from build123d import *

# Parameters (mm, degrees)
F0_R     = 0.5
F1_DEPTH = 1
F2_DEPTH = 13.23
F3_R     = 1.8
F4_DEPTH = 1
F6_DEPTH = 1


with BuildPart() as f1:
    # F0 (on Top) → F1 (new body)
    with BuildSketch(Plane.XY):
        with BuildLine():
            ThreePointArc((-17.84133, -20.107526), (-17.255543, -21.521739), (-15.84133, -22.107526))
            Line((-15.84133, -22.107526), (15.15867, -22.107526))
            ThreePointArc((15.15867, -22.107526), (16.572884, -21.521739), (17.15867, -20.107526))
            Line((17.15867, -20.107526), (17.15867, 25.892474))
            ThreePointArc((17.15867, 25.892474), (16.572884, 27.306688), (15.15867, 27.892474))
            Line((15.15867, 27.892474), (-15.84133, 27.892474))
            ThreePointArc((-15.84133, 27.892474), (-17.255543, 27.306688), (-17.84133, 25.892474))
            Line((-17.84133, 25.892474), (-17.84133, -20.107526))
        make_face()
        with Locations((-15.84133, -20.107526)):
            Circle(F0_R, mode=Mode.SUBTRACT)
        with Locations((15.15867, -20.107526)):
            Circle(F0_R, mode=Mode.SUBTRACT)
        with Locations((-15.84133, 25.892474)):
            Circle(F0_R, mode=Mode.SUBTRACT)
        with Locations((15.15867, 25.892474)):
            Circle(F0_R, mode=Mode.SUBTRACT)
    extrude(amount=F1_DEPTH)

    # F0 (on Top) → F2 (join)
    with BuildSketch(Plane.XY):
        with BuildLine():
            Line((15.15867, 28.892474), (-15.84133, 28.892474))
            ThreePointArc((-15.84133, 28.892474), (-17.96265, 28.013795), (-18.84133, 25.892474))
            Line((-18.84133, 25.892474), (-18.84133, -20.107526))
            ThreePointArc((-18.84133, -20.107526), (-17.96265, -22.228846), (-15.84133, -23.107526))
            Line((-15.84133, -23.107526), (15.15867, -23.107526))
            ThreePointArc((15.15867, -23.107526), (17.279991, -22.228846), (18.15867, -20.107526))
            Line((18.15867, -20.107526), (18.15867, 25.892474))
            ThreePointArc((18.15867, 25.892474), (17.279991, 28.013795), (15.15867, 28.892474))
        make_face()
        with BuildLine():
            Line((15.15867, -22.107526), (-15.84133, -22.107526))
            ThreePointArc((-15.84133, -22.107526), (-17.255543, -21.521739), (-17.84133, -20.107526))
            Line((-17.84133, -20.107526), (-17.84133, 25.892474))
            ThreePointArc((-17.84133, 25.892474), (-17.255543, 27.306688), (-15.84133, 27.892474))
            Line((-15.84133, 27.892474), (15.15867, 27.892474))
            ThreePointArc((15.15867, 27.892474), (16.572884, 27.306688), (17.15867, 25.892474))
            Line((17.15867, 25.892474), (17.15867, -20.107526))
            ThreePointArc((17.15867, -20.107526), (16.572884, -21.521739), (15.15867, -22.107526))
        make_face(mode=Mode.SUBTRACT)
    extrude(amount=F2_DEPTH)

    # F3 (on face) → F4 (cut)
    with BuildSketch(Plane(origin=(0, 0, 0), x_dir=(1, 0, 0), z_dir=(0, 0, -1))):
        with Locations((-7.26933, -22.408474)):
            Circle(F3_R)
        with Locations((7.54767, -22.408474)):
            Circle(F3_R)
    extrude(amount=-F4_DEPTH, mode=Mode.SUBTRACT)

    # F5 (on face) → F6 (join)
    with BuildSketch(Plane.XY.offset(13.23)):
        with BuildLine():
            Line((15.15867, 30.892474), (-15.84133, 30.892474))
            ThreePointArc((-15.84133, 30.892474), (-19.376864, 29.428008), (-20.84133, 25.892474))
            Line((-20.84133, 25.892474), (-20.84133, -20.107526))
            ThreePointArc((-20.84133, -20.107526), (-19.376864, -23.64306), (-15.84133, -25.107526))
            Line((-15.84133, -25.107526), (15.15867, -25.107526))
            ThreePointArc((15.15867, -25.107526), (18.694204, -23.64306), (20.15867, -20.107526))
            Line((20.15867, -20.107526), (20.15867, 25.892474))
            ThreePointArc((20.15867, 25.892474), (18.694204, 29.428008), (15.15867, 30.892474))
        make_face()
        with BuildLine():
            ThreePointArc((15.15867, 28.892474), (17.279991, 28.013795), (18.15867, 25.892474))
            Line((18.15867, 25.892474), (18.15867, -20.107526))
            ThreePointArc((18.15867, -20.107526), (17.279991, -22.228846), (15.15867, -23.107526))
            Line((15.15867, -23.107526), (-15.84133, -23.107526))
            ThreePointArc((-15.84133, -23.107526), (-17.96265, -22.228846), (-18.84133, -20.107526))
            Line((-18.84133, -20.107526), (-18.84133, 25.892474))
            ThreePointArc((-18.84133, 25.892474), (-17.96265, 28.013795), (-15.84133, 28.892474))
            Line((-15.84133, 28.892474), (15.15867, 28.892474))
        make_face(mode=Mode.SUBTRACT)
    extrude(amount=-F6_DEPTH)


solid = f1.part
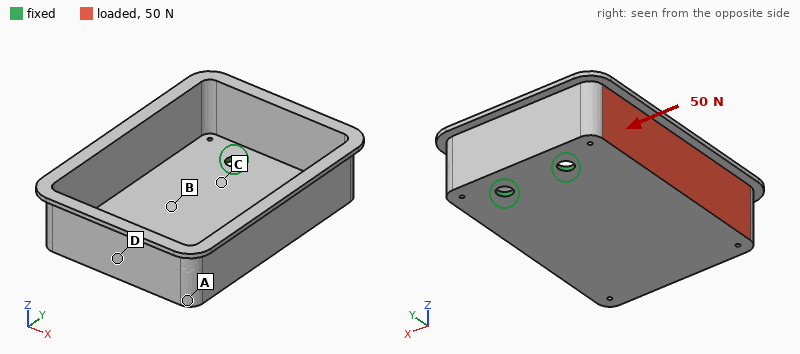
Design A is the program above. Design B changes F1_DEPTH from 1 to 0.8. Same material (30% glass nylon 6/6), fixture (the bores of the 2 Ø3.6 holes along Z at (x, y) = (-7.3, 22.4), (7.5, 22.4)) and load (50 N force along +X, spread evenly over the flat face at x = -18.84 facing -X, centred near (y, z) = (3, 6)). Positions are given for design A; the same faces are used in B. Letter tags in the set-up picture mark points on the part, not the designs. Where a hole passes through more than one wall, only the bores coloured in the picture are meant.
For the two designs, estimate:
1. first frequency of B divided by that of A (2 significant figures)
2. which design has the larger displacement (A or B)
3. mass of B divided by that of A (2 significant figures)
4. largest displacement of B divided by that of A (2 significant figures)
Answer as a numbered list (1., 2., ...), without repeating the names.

1. 0.78
2. B
3. 0.92
4. 1.2
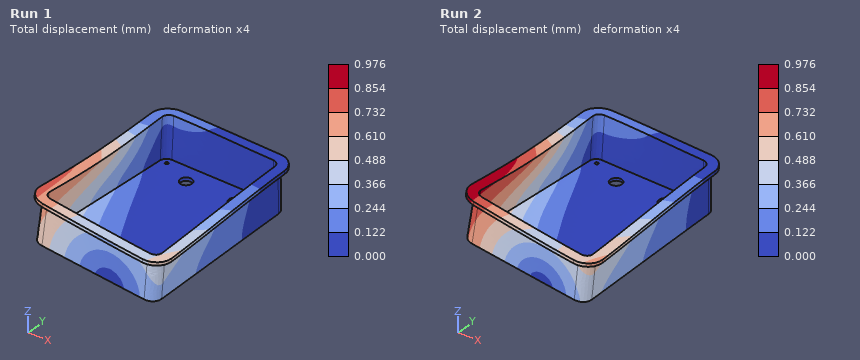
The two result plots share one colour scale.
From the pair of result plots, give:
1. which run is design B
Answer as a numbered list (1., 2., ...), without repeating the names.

1. Run 2
